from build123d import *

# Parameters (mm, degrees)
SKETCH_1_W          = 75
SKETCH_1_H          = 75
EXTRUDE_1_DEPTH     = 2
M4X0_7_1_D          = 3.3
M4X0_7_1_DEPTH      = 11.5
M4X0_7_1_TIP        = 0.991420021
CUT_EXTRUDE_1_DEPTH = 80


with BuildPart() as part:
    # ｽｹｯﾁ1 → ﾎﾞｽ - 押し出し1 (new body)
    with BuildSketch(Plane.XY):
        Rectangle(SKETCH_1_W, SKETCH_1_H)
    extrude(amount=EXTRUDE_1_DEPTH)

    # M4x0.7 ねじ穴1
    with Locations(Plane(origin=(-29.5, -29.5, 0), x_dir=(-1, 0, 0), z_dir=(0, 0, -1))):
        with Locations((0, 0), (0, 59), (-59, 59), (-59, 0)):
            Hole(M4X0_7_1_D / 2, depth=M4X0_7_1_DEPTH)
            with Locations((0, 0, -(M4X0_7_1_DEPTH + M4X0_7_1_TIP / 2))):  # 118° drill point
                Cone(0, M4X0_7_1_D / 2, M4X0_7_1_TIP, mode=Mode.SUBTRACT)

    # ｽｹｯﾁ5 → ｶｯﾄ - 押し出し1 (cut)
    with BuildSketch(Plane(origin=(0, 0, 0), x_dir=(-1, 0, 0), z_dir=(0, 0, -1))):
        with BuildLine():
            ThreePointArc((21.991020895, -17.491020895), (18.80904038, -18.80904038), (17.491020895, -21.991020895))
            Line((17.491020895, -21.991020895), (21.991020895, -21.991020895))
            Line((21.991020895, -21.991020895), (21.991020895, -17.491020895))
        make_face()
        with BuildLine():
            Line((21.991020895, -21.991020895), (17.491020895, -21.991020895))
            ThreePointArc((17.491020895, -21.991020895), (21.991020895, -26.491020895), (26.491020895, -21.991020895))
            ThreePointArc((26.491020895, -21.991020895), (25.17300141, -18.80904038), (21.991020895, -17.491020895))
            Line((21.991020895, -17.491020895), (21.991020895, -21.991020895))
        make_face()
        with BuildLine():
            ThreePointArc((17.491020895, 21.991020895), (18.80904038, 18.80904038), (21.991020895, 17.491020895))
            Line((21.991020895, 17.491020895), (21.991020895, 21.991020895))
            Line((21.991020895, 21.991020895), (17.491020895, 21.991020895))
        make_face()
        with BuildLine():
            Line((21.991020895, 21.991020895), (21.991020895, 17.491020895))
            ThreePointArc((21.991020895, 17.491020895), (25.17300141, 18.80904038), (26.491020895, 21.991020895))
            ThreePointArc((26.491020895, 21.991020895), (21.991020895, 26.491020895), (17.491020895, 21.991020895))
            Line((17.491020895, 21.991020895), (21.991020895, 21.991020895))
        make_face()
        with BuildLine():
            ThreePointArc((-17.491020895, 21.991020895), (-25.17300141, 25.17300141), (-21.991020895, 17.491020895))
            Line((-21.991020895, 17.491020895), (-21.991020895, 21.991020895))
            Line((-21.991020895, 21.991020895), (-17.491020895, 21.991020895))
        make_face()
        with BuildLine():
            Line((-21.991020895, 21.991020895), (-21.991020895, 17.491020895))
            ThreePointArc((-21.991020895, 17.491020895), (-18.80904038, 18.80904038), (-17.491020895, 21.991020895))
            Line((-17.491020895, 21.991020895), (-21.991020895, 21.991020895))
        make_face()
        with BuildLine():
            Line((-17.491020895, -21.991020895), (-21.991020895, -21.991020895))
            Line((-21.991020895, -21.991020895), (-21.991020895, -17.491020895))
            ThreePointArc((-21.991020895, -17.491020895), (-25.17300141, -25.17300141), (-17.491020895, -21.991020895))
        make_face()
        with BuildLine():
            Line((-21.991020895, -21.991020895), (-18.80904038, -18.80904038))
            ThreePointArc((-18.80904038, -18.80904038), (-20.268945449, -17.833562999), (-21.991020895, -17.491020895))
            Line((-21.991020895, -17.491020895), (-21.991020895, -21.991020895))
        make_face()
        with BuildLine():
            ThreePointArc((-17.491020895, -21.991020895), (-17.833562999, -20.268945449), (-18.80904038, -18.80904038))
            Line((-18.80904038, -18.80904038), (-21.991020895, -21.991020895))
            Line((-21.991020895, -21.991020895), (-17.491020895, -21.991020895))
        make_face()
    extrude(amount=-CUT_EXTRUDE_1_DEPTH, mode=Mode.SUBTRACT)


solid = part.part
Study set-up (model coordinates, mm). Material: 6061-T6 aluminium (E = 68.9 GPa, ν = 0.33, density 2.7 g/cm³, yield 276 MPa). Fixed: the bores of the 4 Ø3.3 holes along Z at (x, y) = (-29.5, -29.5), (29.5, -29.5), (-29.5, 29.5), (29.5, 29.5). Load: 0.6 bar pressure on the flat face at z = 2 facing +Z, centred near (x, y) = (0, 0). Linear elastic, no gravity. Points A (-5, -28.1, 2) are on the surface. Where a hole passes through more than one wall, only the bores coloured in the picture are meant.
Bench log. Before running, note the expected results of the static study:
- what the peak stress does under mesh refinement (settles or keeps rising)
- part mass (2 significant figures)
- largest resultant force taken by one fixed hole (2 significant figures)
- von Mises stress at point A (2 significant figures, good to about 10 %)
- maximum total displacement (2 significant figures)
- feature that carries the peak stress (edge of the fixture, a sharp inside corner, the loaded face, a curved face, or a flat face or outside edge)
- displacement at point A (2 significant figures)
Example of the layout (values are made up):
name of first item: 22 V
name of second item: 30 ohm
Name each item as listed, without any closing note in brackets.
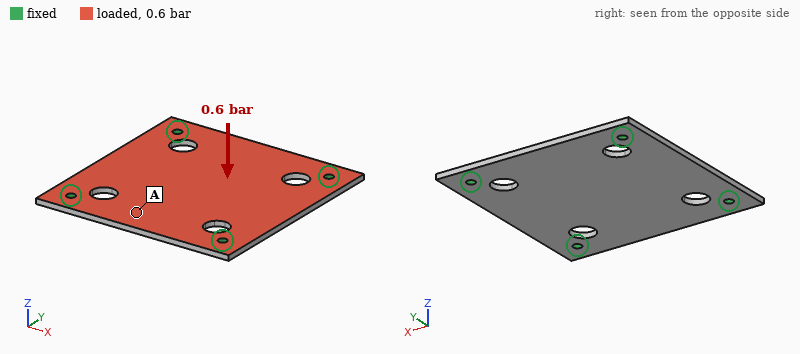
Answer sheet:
what the peak stress does under mesh refinement: keeps rising
part mass: 29 g
largest resultant force taken by one fixed hole: 80 N
von Mises stress at point A: 16 MPa
maximum total displacement: 0.11 mm
feature that carries the peak stress: edge of the fixture
displacement at point A: 0.061 mm
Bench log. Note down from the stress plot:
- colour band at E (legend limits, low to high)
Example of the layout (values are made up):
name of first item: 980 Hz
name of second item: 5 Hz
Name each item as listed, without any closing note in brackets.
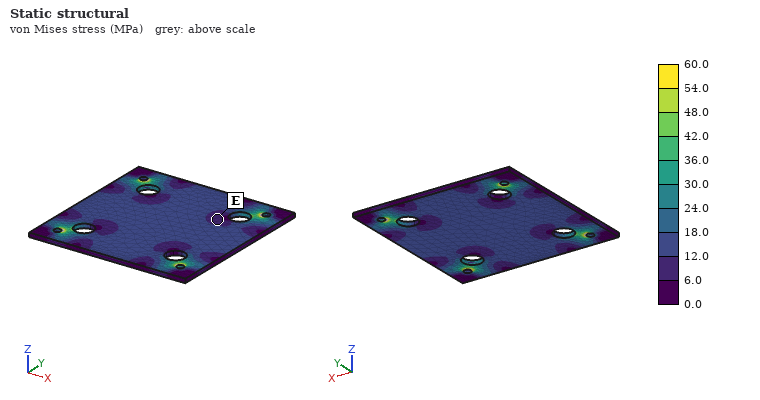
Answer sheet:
colour band at E: 6.0 to 12.0 MPa
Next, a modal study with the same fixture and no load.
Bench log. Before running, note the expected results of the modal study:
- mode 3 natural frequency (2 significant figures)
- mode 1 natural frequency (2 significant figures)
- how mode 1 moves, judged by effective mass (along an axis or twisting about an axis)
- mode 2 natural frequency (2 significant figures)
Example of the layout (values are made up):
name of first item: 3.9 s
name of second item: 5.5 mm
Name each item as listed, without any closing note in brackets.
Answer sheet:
mode 3 natural frequency: 3200 Hz
mode 1 natural frequency: 2000 Hz
how mode 1 moves, judged by effective mass: along Z
mode 2 natural frequency: 3200 Hz
